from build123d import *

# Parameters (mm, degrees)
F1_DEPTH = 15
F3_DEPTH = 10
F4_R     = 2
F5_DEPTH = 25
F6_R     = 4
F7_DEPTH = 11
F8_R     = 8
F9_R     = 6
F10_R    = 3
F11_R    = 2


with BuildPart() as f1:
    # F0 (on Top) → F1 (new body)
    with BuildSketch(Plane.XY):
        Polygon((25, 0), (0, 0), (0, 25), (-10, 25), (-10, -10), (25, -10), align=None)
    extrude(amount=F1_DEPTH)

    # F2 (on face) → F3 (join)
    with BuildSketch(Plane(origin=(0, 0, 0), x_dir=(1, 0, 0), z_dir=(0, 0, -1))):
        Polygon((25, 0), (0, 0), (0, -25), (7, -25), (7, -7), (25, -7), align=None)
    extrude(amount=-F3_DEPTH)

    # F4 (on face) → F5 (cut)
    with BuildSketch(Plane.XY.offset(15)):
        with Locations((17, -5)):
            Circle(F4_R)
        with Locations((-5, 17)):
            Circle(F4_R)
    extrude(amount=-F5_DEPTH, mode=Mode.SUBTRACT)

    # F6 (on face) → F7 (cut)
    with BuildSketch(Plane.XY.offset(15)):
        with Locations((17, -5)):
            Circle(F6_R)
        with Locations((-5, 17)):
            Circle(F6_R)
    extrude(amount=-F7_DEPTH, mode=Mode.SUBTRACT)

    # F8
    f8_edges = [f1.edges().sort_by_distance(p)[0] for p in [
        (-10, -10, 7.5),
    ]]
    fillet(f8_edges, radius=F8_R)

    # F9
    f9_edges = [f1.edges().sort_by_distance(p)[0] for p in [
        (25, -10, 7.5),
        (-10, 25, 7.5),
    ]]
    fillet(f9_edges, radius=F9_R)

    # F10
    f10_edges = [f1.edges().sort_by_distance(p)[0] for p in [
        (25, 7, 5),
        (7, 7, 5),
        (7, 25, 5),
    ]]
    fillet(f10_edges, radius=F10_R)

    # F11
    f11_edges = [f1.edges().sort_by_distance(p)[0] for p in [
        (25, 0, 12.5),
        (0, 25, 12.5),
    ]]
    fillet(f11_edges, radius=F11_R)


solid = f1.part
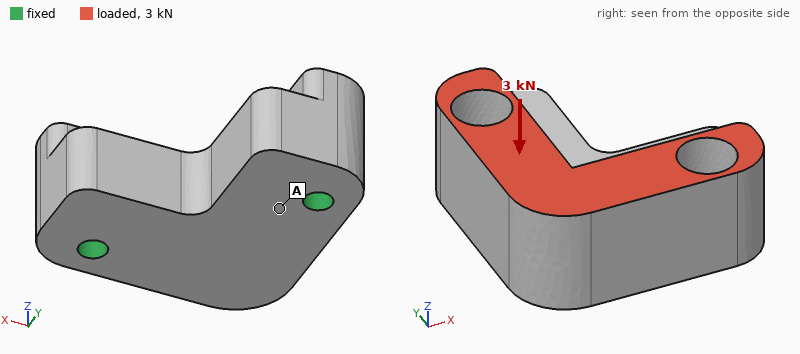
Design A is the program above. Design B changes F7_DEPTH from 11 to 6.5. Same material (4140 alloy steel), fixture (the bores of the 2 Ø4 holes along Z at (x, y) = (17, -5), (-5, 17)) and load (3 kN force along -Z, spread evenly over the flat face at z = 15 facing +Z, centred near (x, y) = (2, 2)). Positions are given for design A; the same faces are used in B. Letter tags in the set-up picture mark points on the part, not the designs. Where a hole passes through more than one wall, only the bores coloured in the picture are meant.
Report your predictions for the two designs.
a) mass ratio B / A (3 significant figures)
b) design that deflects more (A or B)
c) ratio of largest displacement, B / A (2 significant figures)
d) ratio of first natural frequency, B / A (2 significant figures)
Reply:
1.03
A
0.37
1.9
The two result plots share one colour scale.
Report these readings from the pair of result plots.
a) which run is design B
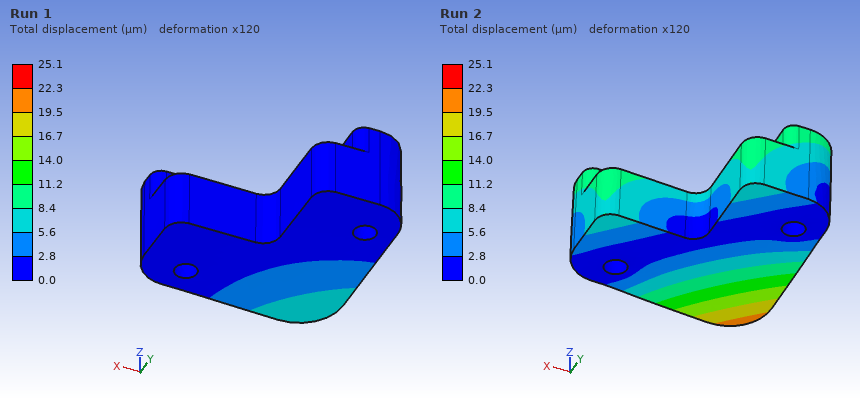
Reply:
Run 1
